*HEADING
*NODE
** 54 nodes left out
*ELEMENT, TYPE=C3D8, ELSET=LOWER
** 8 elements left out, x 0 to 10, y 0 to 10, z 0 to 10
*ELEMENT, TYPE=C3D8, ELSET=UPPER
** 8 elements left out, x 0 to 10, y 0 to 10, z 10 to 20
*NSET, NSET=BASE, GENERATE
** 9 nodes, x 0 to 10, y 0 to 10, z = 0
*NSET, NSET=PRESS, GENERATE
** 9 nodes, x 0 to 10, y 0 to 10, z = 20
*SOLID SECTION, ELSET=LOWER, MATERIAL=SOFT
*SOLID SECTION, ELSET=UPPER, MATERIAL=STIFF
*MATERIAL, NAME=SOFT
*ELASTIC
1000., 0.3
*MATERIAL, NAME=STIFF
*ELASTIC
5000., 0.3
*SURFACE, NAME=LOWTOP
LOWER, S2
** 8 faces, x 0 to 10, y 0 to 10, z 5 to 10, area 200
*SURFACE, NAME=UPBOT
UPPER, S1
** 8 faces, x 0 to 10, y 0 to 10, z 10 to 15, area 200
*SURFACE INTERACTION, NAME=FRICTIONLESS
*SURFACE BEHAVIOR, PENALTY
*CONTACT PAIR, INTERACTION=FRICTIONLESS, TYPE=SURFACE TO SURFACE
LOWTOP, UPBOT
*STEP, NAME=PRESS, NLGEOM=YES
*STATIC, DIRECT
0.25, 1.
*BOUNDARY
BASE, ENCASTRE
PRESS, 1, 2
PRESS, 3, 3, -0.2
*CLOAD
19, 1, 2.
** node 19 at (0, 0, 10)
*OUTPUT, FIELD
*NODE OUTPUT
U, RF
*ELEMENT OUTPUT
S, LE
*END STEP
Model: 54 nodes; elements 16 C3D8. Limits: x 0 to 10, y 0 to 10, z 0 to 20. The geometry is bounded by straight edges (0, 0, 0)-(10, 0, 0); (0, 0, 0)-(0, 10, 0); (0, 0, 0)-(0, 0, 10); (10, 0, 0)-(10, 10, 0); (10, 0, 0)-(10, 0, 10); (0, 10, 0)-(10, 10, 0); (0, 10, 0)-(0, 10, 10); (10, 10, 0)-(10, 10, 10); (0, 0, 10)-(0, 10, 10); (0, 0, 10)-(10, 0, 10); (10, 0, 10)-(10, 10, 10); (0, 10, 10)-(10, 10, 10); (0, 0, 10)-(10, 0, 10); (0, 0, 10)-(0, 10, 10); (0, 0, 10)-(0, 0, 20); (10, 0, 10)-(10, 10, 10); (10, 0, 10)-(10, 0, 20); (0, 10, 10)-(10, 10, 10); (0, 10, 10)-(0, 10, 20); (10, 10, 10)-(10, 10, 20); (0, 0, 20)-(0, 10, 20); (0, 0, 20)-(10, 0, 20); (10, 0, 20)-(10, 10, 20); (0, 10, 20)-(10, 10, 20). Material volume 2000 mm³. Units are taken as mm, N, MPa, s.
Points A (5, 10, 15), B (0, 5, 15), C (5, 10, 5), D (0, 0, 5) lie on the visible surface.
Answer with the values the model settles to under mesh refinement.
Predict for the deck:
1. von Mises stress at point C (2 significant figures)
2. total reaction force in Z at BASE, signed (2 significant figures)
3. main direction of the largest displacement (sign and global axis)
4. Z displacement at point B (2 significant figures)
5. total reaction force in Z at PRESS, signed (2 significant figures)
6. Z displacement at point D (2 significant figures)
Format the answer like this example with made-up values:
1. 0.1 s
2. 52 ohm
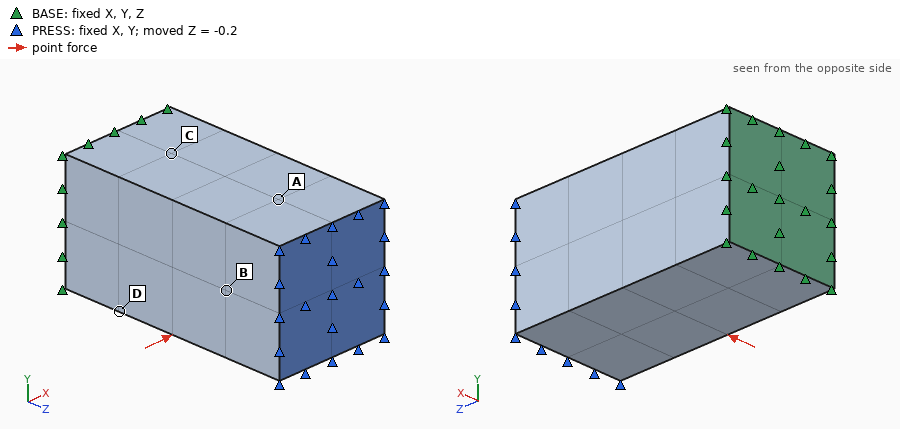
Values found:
1. 17 MPa
2. 1700 N
3. -Z
4. -0.18 mm
5. -1700 N
6. -0.084 mm
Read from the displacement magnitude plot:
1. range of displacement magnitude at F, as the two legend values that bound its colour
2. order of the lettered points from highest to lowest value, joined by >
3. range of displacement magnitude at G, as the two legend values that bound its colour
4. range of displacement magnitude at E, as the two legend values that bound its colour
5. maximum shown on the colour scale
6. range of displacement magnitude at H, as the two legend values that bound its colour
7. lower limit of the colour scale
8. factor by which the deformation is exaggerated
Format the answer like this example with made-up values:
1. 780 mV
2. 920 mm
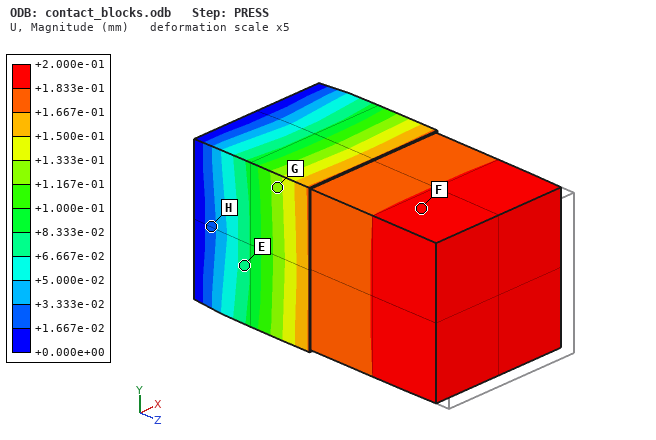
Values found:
1. +1.833e-01 to +2.000e-01 mm
2. F > G > E > H
3. +1.167e-01 to +1.333e-01 mm
4. +6.667e-02 to +8.333e-02 mm
5. +2.000e-01 mm
6. +1.667e-02 to +3.333e-02 mm
7. +0.000e+00 mm
8. 5
